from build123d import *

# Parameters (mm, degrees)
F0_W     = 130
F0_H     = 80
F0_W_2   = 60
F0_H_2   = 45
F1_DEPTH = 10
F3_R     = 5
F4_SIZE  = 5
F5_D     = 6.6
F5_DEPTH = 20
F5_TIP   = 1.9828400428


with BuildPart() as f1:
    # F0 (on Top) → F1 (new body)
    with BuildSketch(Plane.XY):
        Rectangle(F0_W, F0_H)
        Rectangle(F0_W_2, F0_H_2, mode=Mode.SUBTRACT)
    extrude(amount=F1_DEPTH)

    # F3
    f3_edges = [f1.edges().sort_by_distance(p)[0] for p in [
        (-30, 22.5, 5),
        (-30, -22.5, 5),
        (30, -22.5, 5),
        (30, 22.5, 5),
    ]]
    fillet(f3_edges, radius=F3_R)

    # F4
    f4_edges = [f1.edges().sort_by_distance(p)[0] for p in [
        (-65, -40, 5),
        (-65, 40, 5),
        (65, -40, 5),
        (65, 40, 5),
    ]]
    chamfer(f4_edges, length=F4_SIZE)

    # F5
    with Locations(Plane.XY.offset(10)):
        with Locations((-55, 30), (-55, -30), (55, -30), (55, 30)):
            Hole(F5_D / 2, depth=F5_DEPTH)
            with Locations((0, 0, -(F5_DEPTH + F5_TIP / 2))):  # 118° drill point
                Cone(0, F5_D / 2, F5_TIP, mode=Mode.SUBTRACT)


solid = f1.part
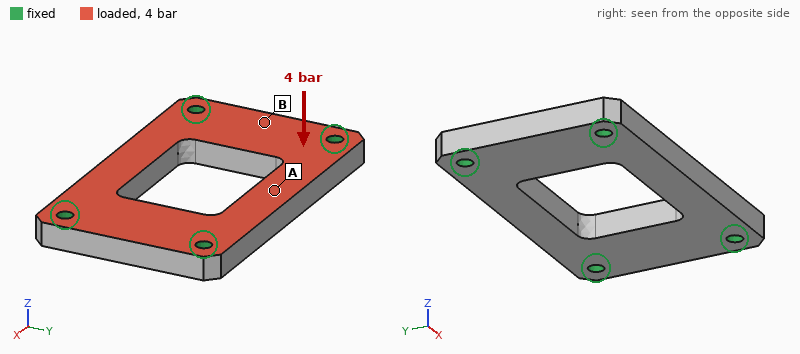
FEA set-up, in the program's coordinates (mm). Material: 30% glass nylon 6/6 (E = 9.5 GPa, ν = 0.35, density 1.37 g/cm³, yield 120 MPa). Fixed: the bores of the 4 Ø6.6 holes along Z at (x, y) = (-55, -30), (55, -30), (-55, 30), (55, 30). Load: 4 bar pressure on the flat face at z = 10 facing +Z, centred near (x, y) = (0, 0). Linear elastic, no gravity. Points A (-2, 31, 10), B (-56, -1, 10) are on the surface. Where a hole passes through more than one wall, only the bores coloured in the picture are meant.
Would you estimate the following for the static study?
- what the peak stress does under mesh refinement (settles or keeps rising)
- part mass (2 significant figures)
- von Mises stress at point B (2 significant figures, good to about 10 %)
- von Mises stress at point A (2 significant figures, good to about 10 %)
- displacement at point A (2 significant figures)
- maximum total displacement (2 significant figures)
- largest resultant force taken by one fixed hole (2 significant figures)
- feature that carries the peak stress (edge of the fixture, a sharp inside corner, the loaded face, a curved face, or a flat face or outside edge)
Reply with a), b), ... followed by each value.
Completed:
a) keeps rising
b) 100 g
c) 3.5 MPa
d) 11 MPa
e) 0.19 mm
f) 0.20 mm
g) 750 N
h) edge of the fixture
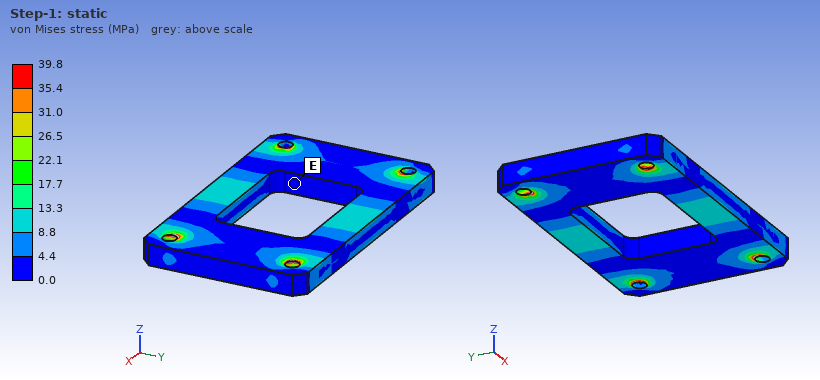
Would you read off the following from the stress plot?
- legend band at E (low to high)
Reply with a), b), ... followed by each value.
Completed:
a) 0.0 to 4.4 MPa
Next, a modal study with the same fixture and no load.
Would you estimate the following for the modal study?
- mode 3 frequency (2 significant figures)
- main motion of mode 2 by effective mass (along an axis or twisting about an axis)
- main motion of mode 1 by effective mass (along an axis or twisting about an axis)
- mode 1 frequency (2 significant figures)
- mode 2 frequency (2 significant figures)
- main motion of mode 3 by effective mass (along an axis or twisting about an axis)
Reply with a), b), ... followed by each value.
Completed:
a) 4700 Hz
b) twisting about X
c) along Z
d) 2300 Hz
e) 2600 Hz
f) twisting about Y
